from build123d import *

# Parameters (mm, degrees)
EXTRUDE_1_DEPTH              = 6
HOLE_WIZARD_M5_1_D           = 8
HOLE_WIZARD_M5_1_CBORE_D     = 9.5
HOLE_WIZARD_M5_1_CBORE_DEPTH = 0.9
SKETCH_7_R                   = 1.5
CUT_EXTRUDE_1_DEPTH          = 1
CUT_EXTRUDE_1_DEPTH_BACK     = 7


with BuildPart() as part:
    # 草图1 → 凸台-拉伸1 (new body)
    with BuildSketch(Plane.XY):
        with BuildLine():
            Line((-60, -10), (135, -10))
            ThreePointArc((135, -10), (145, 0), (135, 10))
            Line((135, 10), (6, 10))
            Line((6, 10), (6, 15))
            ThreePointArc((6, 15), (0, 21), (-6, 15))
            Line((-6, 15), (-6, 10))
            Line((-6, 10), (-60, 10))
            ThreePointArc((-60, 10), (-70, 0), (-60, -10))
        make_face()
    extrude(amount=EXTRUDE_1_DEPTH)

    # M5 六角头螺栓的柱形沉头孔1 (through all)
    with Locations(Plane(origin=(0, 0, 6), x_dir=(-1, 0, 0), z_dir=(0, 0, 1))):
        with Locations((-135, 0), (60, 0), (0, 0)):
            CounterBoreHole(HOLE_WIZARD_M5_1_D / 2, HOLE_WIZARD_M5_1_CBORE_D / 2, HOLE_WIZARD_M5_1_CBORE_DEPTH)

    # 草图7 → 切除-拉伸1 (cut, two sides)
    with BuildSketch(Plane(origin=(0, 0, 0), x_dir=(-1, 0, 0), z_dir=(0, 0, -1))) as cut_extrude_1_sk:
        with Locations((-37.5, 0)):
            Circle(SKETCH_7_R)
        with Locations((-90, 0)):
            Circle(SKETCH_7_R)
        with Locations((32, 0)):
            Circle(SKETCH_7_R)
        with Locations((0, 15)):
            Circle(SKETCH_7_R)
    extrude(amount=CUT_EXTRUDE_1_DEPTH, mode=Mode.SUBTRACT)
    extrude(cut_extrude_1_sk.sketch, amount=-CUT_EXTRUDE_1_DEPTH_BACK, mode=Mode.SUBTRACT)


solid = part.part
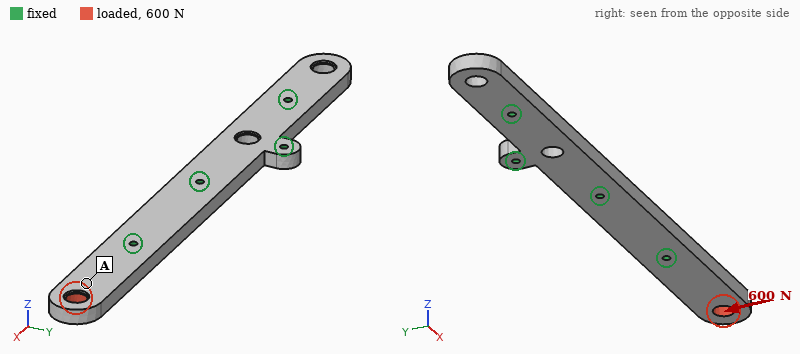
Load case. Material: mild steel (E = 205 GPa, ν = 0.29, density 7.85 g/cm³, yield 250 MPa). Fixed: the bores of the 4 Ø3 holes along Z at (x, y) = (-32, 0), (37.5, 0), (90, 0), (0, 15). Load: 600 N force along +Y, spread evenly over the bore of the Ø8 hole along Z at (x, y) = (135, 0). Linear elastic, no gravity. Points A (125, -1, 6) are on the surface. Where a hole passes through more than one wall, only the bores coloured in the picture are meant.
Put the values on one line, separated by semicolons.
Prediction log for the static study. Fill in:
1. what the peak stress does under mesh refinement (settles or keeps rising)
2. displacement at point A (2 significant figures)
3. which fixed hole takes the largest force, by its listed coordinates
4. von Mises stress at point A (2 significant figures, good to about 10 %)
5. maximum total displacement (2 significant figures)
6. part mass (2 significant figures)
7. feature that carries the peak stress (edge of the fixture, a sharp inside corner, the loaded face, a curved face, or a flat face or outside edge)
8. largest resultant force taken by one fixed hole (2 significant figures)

keeps rising; 33 µm; (90, 0); 13 MPa; 59 µm; 200 g; edge of the fixture; 1.1 kN
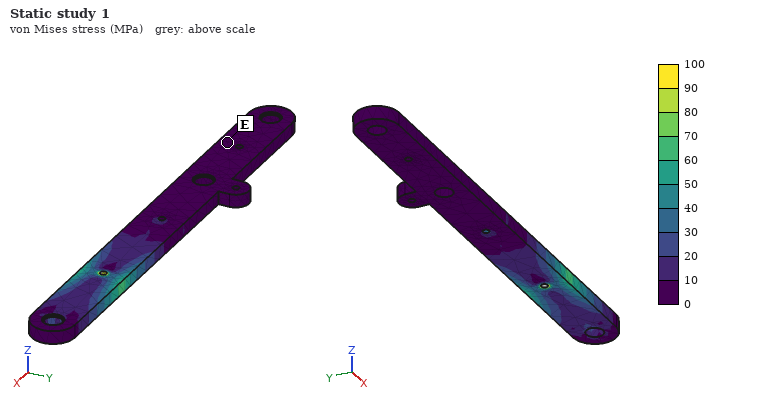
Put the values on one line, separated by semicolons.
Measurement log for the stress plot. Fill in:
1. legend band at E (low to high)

0 to 10 MPa
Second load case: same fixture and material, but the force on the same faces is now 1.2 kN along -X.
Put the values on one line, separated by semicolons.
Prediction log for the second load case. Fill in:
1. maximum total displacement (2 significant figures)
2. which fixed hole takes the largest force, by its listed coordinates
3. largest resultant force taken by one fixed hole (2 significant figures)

12 µm; (90, 0); 1.1 kN
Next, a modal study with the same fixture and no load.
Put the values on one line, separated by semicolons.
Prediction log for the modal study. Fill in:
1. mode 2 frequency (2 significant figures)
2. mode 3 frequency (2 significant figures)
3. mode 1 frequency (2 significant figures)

3800 Hz; 4100 Hz; 1800 Hz
